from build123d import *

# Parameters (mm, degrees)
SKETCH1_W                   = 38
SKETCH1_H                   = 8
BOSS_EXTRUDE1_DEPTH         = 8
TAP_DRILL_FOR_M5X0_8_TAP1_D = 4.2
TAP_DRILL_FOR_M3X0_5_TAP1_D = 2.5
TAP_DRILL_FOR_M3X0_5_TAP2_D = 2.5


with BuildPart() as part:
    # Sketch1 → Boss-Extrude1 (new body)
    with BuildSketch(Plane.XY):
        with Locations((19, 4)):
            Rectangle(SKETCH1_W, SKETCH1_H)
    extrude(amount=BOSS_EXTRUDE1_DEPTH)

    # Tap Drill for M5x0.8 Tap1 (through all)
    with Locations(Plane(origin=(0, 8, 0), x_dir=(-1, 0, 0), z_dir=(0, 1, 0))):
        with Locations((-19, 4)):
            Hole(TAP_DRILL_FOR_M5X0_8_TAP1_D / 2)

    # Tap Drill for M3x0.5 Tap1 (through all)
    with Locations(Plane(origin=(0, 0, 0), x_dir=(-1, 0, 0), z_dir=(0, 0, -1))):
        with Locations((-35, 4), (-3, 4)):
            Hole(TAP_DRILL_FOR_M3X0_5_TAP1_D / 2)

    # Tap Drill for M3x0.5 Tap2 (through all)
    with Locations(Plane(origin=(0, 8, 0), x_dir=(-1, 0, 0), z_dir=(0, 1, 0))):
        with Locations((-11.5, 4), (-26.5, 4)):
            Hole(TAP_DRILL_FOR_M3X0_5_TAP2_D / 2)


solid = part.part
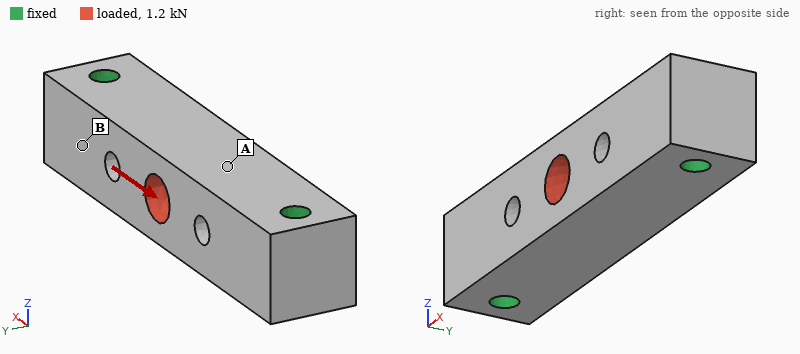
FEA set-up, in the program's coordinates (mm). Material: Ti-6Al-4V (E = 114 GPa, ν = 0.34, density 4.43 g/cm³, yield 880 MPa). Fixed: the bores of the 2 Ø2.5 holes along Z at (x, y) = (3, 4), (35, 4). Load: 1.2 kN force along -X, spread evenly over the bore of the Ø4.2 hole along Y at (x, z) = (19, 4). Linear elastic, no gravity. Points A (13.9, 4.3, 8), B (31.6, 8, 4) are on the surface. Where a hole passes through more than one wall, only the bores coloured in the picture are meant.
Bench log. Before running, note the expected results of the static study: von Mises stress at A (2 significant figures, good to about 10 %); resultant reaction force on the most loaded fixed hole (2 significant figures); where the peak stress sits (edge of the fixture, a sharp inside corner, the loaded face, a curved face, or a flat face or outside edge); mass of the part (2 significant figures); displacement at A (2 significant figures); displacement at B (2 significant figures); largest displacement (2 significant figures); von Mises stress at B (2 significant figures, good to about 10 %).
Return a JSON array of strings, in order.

["11 MPa", "600 N", "a curved face", "9.6 g", "1.1 µm", "0.38 µm", "1.6 µm", "4.6 MPa"]
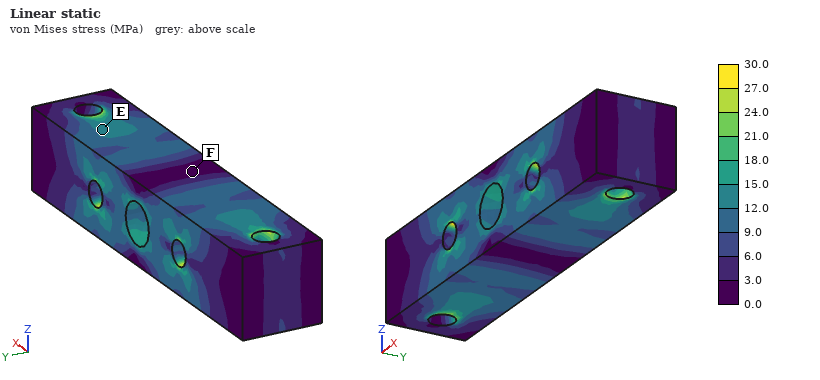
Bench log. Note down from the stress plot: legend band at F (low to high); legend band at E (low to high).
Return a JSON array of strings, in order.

["0.0 to 3.0 MPa", "12.0 to 15.0 MPa"]
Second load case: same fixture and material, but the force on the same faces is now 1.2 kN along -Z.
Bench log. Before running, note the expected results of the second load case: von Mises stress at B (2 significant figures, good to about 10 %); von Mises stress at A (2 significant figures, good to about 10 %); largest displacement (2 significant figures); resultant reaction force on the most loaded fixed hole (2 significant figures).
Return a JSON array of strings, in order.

["21 MPa", "29 MPa", "10 µm", "600 N"]
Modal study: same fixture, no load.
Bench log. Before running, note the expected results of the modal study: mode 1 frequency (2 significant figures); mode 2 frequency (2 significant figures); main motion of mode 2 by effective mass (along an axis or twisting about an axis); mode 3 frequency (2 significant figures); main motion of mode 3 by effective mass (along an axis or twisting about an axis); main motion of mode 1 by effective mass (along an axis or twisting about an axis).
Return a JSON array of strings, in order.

["25 kHz", "31 kHz", "along Z", "45 kHz", "twisting about X", "along Y"]
